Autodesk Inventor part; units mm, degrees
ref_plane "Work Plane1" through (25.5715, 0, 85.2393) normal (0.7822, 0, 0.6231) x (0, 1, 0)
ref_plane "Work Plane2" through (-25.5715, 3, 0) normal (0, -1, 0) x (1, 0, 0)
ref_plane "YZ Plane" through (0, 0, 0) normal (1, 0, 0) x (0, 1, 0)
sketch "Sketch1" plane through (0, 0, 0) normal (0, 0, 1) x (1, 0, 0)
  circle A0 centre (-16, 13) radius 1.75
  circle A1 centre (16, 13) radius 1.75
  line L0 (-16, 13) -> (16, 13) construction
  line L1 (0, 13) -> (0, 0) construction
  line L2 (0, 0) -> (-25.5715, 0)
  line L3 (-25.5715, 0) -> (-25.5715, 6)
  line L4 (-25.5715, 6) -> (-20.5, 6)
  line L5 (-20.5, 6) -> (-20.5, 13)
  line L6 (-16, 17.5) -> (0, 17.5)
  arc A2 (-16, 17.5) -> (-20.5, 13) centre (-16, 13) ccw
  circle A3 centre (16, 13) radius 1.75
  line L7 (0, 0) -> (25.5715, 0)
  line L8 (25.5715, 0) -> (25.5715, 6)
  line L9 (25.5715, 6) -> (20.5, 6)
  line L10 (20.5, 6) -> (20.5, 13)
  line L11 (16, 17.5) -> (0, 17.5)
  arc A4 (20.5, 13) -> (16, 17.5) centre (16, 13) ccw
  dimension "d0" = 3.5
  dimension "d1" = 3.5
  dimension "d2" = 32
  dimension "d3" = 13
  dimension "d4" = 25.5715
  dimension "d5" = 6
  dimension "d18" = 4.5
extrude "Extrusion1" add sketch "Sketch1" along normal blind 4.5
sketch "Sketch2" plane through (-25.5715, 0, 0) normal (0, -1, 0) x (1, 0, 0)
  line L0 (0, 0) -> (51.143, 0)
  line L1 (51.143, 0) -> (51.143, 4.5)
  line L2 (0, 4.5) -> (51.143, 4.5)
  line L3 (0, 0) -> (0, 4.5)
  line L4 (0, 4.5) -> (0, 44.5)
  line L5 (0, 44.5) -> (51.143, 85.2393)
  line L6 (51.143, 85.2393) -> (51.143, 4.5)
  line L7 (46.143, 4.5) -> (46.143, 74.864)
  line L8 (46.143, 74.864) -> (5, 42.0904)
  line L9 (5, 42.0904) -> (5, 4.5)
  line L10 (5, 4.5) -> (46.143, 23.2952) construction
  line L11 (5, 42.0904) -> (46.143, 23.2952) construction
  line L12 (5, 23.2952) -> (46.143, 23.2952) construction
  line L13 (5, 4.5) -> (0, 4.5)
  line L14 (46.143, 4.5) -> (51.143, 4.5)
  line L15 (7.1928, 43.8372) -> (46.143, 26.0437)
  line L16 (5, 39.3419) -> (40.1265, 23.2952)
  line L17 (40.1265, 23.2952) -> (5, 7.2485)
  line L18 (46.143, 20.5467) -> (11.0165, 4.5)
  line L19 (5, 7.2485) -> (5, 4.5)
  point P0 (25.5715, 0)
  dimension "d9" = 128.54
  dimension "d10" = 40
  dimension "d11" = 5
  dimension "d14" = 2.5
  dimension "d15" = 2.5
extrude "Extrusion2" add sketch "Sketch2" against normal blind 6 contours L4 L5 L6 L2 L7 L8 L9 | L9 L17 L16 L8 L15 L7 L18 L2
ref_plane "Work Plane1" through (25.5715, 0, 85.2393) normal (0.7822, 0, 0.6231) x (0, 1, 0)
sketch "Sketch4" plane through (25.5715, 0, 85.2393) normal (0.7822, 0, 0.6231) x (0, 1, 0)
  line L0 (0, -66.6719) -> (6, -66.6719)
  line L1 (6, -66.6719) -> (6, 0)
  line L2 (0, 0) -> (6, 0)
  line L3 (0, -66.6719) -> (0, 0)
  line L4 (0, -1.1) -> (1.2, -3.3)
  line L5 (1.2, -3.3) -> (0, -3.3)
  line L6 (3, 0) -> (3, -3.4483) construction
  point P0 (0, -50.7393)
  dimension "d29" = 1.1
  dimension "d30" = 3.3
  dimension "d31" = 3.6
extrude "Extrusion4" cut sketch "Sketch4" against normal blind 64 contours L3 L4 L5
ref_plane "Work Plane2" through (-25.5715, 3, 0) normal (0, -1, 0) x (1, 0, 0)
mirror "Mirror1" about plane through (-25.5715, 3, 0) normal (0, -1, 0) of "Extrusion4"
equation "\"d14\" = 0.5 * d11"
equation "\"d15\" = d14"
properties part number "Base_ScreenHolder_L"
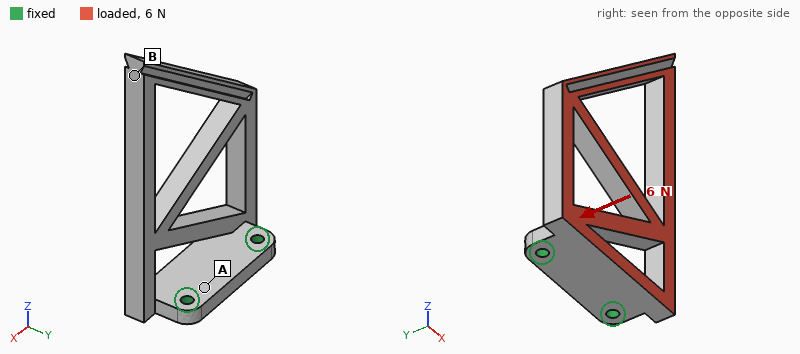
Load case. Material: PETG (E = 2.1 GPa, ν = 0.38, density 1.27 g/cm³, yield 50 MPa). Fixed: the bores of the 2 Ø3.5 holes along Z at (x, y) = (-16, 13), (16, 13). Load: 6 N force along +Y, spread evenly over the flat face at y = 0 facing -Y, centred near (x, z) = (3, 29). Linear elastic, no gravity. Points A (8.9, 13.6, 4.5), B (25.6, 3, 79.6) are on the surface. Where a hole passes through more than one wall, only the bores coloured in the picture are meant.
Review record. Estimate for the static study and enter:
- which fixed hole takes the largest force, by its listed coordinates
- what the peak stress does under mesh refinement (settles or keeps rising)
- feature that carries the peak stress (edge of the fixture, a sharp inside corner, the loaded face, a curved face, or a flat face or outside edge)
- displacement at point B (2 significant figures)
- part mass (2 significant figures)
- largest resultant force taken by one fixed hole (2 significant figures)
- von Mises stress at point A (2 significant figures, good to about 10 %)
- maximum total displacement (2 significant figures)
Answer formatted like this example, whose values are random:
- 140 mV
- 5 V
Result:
- (16, 13)
- keeps rising
- a sharp inside corner
- 0.93 mm
- 14 g
- 3.4 N
- 0.46 MPa
- 1.0 mm
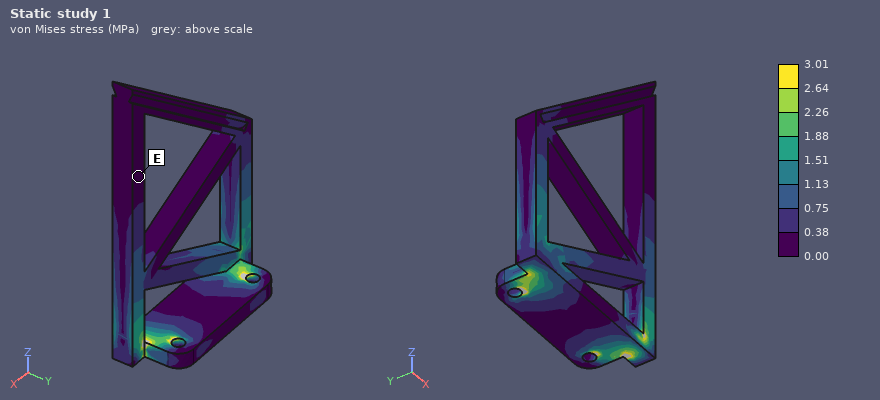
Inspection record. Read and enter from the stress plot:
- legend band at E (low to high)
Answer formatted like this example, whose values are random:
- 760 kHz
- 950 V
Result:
- 0.00 to 0.38 MPa
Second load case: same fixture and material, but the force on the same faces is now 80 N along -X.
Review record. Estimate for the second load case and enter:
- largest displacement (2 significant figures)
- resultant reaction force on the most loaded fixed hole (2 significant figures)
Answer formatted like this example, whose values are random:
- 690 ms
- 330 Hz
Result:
- 0.71 mm
- 80 N
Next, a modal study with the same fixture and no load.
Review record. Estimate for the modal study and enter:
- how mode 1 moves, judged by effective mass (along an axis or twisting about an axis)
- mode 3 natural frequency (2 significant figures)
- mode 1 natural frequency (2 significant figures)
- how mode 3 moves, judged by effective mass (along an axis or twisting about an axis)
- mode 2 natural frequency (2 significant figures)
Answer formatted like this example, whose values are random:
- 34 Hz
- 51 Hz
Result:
- along Y
- 610 Hz
- 150 Hz
- along X
- 490 Hz
